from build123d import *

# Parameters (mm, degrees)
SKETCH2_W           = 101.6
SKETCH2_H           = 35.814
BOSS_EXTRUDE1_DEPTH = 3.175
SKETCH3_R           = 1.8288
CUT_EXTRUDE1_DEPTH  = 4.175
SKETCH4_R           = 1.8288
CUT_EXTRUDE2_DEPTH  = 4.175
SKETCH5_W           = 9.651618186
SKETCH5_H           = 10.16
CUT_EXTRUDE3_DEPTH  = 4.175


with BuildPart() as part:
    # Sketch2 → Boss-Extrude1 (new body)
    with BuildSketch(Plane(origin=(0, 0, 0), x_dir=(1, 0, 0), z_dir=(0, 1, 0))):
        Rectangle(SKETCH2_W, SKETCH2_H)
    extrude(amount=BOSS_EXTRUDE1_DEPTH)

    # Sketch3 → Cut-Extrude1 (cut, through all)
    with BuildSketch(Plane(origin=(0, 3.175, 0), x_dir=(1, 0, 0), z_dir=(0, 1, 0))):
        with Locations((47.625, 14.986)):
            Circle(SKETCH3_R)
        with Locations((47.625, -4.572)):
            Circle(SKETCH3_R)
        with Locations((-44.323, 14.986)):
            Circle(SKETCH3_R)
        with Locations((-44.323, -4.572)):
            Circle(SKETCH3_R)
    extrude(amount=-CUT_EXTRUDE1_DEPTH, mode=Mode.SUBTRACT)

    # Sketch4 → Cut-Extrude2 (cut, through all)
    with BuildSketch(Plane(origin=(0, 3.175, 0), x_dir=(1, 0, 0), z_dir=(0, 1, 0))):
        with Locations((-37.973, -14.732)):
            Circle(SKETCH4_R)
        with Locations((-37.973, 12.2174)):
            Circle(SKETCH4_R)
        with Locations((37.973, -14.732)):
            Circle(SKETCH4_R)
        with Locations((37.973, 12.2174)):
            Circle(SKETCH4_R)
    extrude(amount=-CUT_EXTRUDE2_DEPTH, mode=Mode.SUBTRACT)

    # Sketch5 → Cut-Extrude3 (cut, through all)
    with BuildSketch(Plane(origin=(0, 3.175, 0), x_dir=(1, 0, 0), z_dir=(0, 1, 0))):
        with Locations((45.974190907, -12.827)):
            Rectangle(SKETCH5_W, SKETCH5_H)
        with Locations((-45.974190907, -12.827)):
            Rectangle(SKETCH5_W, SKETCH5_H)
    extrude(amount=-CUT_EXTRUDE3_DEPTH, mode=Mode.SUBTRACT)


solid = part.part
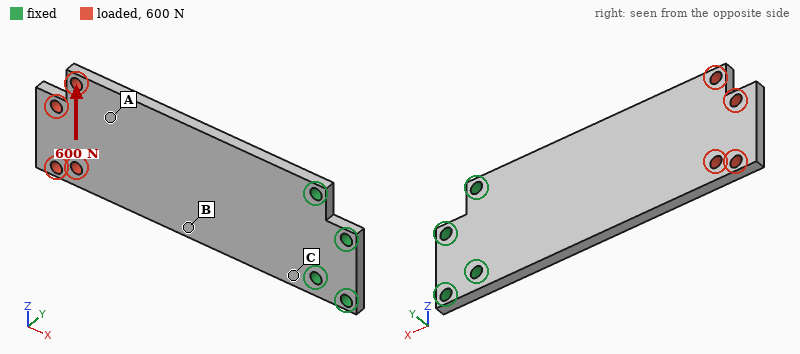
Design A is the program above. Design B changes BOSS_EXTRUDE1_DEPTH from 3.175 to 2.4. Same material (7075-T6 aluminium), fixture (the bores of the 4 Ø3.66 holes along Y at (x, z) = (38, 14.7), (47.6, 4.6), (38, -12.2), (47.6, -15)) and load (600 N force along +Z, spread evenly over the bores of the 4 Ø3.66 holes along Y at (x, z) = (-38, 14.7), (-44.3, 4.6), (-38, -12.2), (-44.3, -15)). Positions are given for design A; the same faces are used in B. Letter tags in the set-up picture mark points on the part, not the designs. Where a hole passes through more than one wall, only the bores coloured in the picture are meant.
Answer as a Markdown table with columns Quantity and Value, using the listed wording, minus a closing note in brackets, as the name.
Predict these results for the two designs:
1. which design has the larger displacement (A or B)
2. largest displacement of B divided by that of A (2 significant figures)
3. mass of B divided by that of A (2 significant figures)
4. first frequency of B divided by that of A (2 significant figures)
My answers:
| Quantity | Value |
|---|---|
| which design has the larger displacement | B |
| largest displacement of B divided by that of A | 1.3 |
| mass of B divided by that of A | 0.76 |
| first frequency of B divided by that of A | 0.76 |
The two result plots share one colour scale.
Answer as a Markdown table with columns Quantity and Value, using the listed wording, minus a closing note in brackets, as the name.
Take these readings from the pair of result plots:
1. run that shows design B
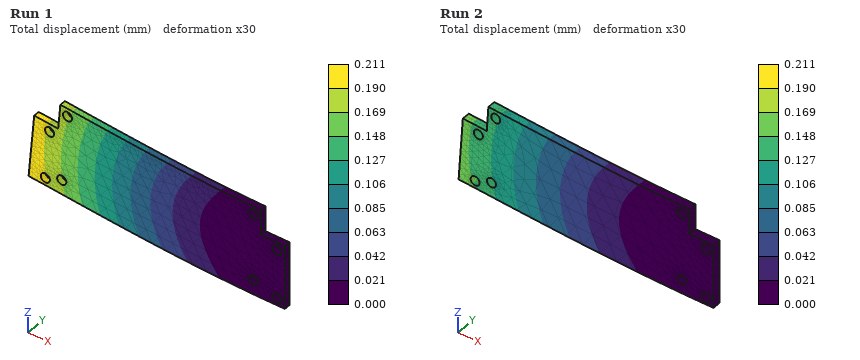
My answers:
| Quantity | Value |
|---|---|
| run that shows design B | Run 1 |
